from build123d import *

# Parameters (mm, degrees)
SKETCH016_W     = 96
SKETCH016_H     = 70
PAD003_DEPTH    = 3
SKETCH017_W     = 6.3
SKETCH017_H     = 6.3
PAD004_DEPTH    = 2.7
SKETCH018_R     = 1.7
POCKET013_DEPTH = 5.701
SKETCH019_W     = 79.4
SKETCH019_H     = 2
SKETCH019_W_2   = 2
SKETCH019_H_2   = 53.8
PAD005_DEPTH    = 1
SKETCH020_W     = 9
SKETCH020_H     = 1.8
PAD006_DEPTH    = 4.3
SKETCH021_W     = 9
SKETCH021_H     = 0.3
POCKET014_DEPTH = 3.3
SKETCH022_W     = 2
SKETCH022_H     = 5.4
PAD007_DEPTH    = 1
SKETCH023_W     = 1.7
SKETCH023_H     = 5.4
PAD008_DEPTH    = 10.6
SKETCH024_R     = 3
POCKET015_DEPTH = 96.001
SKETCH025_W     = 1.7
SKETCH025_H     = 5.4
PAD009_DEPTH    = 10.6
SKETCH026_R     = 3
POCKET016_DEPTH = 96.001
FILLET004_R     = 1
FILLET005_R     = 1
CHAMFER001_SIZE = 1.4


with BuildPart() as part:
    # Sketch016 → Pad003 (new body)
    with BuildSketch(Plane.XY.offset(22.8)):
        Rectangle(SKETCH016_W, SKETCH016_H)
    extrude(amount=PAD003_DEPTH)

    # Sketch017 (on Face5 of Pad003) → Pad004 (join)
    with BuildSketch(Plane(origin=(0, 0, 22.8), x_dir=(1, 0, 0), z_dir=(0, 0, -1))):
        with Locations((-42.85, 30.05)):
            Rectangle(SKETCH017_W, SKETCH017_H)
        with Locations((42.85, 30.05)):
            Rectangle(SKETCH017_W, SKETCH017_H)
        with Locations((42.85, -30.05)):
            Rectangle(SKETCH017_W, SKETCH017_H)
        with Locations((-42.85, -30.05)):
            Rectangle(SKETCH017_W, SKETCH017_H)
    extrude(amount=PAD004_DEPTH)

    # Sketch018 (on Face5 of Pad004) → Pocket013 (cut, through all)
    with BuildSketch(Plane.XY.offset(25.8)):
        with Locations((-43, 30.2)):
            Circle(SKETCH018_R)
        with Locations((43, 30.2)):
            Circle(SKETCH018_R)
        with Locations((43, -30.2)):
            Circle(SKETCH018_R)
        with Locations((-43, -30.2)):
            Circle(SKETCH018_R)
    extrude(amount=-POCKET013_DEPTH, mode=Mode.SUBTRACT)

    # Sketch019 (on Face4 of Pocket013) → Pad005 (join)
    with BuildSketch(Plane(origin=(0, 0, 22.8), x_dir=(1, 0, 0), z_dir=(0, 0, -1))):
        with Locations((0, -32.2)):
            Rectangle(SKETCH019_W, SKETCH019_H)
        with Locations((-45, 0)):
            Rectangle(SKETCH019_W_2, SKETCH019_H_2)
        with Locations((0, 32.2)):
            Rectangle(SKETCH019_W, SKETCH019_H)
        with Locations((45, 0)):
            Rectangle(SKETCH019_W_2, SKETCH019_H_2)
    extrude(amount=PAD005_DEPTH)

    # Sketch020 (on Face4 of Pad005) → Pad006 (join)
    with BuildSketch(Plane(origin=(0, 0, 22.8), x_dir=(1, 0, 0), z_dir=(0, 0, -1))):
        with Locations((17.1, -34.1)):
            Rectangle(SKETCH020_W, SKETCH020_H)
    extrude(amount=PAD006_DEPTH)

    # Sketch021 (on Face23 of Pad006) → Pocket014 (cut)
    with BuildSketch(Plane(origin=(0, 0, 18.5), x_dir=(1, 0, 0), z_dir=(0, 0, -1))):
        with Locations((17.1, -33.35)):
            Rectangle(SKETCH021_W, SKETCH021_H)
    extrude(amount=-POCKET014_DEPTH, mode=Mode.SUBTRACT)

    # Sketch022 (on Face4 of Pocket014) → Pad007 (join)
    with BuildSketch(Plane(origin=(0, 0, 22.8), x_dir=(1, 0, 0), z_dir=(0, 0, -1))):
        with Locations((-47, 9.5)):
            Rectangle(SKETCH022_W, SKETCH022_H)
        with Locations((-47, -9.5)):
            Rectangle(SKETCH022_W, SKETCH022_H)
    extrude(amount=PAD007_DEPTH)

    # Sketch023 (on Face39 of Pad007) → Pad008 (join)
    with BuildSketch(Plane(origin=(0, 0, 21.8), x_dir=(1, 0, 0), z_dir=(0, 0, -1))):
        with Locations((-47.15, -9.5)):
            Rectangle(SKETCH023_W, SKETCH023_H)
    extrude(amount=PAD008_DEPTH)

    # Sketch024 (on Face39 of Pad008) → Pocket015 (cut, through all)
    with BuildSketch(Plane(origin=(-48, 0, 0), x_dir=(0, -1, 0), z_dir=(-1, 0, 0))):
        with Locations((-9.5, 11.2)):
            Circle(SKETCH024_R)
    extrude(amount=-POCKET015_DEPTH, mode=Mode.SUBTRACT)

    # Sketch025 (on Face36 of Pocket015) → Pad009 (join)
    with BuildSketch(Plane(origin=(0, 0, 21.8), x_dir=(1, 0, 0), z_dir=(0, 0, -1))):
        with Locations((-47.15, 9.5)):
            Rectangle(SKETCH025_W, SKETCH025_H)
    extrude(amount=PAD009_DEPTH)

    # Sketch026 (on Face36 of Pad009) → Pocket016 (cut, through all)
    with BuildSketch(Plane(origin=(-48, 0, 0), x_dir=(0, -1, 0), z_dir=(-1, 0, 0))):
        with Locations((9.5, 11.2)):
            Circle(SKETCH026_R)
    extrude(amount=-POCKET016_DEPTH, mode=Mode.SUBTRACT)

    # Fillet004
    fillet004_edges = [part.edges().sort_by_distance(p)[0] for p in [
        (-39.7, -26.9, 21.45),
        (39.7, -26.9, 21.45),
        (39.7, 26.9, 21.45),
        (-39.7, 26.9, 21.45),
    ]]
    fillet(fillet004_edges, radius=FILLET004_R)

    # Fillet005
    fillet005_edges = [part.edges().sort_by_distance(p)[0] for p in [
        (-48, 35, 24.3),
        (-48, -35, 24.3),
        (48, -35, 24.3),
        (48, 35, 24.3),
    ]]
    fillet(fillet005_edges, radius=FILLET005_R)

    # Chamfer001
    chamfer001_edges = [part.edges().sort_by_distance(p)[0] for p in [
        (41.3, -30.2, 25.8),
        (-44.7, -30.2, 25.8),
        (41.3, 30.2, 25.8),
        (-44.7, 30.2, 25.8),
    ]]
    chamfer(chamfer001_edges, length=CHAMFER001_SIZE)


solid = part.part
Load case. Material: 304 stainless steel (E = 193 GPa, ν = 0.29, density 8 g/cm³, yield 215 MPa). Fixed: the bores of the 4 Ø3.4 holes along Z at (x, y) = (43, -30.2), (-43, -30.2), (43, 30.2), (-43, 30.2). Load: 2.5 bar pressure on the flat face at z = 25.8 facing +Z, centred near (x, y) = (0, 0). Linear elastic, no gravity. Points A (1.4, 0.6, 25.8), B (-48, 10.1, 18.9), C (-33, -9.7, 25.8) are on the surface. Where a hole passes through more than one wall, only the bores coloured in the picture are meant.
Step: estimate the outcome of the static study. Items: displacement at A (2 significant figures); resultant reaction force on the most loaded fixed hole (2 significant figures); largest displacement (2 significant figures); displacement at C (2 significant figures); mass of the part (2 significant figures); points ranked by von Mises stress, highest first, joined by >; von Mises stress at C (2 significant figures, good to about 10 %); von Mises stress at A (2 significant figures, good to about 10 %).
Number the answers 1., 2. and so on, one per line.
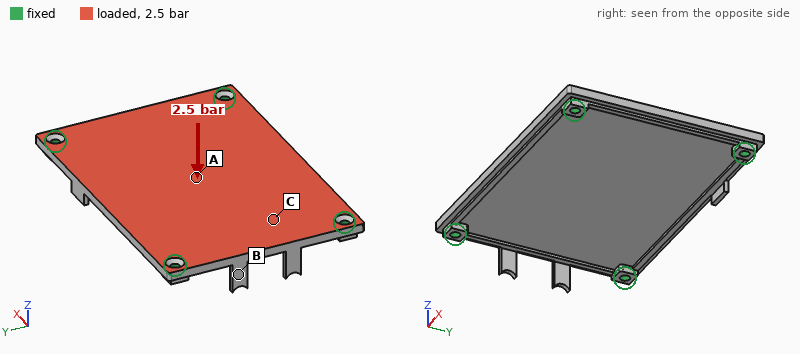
1. 0.12 mm
2. 610 N
3. 0.12 mm
4. 0.050 mm
5. 170 g
6. A > C > B
7. 31 MPa
8. 54 MPa
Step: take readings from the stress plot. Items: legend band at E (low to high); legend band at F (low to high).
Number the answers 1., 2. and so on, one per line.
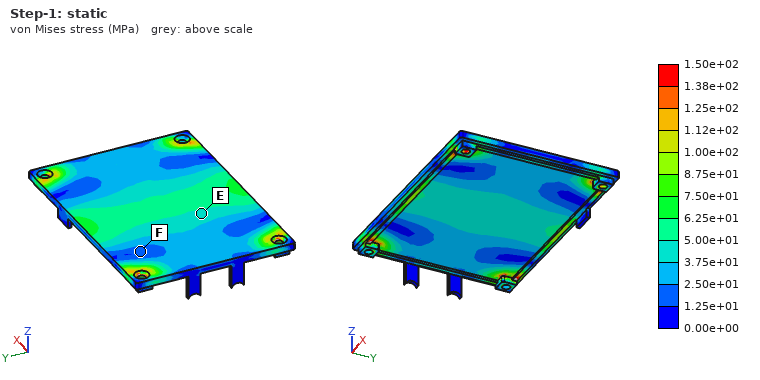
1. 3.75e+01 to 5.00e+01 MPa
2. 1.25e+01 to 2.50e+01 MPa
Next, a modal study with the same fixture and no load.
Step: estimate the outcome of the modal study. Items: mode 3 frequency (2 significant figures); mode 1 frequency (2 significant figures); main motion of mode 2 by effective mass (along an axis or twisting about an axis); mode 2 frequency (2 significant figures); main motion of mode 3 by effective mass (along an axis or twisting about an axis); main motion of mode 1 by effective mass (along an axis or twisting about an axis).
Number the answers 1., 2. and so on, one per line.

1. 3900 Hz
2. 1700 Hz
3. twisting about X
4. 2800 Hz
5. twisting about Y
6. along Z
